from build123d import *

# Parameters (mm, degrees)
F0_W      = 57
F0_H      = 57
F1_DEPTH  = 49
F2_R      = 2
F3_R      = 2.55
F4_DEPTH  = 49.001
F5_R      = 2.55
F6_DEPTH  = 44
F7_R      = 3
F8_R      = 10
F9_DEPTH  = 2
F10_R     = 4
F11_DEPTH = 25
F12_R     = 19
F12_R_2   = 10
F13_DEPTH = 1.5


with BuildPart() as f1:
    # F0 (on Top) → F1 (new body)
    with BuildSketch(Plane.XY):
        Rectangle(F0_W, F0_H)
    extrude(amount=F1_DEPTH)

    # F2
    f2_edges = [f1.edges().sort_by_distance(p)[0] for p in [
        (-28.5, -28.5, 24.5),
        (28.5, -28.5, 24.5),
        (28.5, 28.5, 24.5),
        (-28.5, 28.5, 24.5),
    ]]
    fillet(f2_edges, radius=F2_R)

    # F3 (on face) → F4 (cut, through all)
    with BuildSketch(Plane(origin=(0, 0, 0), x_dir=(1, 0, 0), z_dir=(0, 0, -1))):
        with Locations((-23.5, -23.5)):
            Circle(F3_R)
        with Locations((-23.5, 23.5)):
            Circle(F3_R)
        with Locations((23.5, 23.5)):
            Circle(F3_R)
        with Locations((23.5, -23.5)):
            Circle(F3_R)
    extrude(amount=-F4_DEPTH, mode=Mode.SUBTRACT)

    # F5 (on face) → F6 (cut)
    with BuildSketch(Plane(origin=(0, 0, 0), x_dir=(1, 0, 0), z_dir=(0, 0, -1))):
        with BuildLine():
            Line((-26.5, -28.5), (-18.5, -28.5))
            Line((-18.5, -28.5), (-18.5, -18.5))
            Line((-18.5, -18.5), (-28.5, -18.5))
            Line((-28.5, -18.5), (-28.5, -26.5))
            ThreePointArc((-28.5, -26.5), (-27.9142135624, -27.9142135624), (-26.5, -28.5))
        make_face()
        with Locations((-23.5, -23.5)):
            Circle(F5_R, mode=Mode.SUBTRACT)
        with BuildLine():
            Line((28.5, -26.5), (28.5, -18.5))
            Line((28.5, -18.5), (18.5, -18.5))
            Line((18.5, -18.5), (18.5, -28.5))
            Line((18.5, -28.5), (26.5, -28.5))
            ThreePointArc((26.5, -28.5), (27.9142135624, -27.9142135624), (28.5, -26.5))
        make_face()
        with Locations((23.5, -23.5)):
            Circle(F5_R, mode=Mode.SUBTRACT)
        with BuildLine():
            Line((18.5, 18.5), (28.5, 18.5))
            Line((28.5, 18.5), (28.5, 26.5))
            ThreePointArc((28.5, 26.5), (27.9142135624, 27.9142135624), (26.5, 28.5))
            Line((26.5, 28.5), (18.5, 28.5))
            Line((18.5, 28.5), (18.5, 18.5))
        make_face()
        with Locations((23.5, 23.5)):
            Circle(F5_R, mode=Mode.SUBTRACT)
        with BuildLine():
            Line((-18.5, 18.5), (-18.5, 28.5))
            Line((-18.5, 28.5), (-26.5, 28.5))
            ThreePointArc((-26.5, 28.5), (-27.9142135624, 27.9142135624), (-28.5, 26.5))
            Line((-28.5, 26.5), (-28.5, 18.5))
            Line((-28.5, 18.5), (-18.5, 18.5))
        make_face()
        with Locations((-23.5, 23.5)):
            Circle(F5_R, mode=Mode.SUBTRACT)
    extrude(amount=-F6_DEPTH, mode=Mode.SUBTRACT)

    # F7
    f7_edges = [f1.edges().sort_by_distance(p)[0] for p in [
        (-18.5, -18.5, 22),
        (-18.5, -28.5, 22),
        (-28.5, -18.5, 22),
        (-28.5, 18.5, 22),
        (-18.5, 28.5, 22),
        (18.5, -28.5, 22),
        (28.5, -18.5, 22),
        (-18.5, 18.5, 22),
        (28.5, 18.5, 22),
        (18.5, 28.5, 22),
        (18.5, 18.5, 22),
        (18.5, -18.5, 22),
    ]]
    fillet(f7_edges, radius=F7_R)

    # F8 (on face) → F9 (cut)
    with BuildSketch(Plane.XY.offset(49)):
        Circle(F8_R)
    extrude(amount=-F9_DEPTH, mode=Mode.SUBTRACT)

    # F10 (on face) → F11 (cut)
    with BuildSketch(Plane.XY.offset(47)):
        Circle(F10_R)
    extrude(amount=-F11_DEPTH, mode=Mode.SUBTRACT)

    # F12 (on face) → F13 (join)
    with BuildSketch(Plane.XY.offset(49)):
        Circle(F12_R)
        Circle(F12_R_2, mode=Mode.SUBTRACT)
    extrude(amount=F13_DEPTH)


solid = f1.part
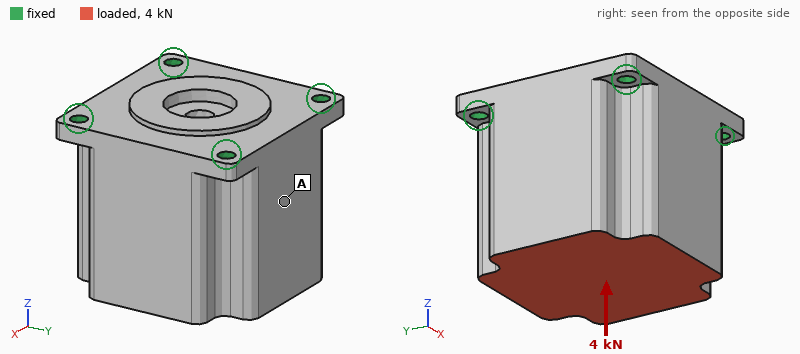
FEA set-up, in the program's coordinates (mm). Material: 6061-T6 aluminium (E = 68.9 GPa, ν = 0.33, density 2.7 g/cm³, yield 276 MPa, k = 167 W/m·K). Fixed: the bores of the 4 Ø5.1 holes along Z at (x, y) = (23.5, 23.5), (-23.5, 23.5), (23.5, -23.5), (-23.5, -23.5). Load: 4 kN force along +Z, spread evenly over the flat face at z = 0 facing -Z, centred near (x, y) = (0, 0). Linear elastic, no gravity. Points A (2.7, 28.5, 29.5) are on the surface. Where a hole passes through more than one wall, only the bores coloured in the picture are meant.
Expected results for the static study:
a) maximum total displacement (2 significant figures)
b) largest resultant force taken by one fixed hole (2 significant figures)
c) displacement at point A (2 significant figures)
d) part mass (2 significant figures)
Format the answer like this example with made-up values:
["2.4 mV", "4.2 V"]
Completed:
["5.3 µm", "1.1 kN", "4.7 µm", "380 g"]
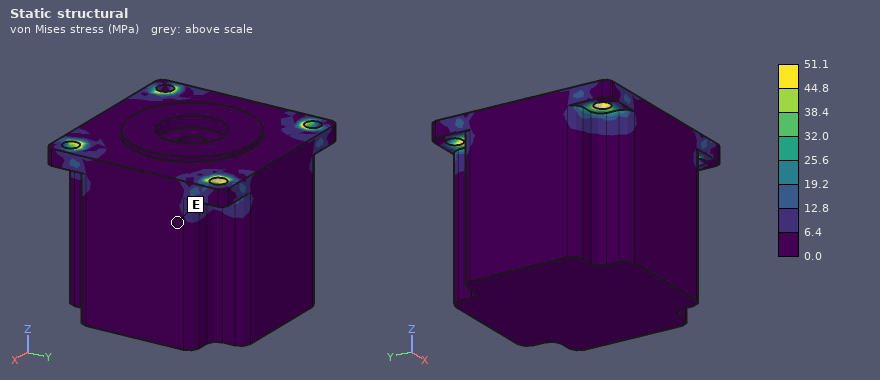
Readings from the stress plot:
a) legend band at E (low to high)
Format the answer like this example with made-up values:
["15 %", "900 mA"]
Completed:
["0.0 to 6.4 MPa"]
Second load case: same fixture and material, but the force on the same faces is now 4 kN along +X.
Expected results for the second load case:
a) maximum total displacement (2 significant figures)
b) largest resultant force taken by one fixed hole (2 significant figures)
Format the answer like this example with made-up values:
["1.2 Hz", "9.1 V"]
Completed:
["29 µm", "2.4 kN"]
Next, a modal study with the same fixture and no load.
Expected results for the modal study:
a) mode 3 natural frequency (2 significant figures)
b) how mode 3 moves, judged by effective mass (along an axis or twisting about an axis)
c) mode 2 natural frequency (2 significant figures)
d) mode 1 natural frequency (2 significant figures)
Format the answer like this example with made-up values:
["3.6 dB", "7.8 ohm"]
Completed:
["7600 Hz", "along Z", "5200 Hz", "5200 Hz"]
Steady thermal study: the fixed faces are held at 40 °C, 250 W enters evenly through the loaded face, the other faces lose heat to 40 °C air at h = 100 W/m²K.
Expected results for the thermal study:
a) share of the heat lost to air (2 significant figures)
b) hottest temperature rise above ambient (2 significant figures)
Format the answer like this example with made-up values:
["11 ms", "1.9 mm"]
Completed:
["18 %", "48 K"]
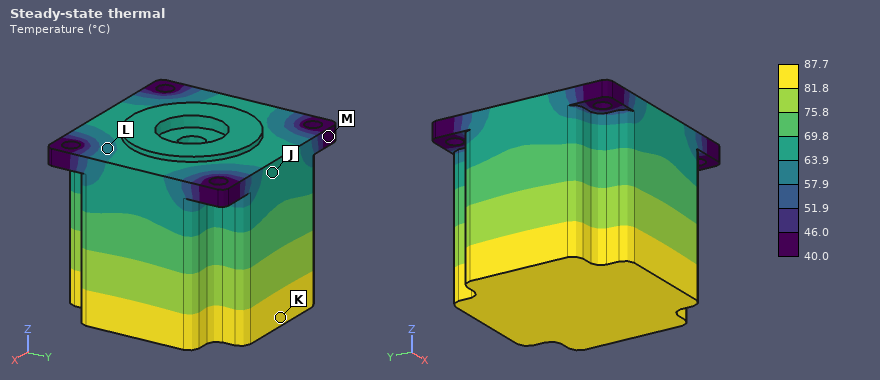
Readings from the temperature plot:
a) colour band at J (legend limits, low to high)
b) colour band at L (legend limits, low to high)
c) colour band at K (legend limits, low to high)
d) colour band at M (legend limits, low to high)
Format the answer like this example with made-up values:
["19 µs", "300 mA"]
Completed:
["63.9 to 69.8 °C", "57.9 to 63.9 °C", "81.8 to 87.7 °C", "40.0 to 46.0 °C"]
